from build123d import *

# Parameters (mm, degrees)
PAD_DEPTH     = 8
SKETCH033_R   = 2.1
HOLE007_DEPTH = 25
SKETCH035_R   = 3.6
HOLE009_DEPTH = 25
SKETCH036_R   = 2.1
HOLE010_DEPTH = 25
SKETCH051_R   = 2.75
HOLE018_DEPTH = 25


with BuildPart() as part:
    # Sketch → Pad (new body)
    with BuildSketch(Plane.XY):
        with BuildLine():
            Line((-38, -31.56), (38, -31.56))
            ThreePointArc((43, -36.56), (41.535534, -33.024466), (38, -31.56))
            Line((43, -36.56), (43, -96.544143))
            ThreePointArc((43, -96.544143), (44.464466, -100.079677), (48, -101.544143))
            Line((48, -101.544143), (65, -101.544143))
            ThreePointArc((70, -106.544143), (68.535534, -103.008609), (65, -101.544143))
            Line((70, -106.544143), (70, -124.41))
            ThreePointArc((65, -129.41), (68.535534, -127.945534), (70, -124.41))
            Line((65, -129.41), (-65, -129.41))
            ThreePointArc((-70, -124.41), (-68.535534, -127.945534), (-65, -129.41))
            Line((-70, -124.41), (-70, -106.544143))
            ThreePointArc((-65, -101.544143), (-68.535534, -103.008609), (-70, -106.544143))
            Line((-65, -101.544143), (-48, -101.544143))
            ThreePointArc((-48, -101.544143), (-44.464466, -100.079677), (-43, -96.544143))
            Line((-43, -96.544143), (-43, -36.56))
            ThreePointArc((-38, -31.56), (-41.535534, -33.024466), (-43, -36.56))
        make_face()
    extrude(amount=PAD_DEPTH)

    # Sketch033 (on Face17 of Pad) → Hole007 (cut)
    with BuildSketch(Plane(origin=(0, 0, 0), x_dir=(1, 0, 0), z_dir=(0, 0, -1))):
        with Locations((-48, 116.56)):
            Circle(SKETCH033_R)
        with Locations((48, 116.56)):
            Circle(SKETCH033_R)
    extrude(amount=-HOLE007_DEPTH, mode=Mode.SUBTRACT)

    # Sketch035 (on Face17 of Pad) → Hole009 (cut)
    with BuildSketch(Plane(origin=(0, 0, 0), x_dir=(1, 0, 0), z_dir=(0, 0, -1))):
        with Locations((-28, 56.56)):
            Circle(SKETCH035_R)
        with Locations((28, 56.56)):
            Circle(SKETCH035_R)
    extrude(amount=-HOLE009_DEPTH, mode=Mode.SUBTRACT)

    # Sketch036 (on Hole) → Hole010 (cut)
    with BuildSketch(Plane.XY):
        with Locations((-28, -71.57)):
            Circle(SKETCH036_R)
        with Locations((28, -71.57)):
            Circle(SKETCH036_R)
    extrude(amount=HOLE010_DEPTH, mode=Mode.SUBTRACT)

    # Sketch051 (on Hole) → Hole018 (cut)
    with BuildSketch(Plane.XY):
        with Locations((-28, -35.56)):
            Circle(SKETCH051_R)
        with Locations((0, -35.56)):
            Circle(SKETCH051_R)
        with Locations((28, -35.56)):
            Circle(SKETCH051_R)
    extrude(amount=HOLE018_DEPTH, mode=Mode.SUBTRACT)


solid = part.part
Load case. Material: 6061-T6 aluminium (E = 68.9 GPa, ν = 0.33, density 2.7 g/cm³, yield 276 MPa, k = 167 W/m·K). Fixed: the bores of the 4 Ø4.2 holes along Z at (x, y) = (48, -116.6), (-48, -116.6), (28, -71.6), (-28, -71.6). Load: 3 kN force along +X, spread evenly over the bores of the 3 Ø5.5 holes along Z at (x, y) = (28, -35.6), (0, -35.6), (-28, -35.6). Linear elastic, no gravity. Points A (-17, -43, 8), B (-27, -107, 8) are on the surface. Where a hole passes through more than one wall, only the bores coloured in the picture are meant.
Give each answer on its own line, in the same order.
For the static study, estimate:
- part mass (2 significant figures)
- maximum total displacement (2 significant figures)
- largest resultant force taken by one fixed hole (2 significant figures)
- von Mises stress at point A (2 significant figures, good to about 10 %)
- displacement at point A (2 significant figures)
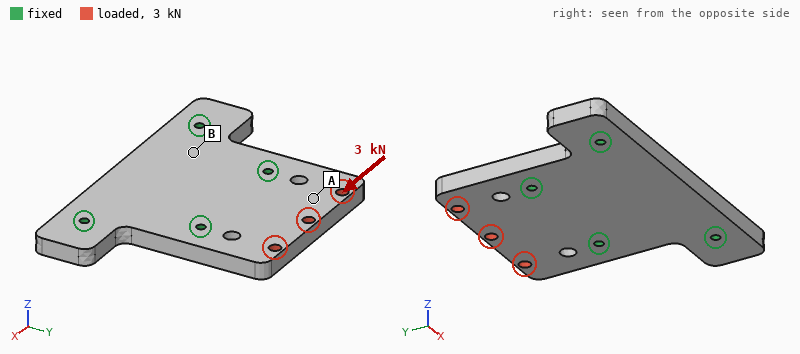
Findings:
210 g
15 µm
2.1 kN
8.7 MPa
9.4 µm
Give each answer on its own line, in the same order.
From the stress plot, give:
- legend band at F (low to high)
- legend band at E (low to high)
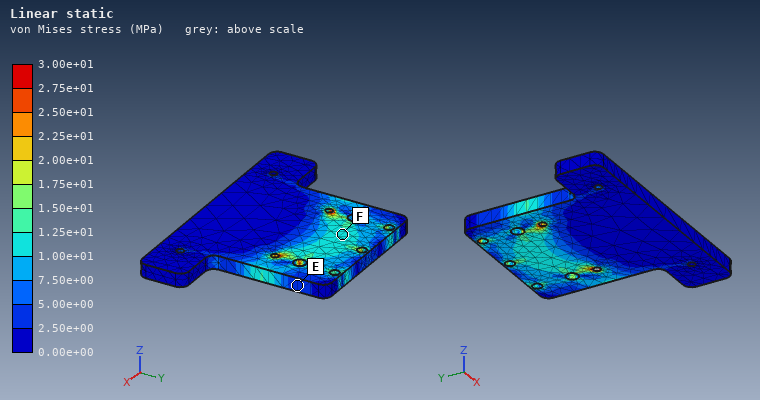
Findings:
1.00e+01 to 1.25e+01 MPa
2.50e+00 to 5.00e+00 MPa
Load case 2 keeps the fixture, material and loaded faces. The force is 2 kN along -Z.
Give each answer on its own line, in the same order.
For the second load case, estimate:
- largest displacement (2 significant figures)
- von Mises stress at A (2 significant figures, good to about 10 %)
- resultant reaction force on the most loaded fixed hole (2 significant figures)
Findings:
0.23 mm
18 MPa
1.3 kN
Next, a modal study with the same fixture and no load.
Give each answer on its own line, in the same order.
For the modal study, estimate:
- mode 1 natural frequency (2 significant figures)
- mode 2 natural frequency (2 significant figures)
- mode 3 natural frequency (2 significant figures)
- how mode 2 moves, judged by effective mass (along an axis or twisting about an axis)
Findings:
3300 Hz
4700 Hz
5300 Hz
along Z
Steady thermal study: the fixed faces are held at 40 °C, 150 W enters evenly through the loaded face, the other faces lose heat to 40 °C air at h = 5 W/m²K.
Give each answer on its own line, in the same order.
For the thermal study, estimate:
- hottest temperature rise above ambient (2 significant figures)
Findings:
73 K
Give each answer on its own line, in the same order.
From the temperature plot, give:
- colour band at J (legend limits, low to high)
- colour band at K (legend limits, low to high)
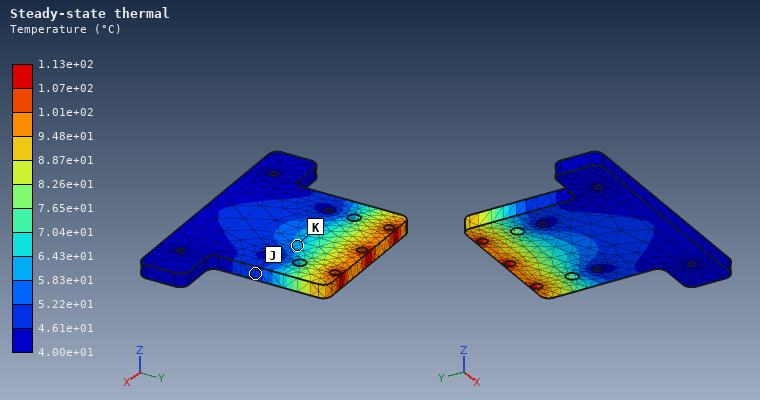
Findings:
4.61e+01 to 5.22e+01 °C
5.83e+01 to 6.43e+01 °C
